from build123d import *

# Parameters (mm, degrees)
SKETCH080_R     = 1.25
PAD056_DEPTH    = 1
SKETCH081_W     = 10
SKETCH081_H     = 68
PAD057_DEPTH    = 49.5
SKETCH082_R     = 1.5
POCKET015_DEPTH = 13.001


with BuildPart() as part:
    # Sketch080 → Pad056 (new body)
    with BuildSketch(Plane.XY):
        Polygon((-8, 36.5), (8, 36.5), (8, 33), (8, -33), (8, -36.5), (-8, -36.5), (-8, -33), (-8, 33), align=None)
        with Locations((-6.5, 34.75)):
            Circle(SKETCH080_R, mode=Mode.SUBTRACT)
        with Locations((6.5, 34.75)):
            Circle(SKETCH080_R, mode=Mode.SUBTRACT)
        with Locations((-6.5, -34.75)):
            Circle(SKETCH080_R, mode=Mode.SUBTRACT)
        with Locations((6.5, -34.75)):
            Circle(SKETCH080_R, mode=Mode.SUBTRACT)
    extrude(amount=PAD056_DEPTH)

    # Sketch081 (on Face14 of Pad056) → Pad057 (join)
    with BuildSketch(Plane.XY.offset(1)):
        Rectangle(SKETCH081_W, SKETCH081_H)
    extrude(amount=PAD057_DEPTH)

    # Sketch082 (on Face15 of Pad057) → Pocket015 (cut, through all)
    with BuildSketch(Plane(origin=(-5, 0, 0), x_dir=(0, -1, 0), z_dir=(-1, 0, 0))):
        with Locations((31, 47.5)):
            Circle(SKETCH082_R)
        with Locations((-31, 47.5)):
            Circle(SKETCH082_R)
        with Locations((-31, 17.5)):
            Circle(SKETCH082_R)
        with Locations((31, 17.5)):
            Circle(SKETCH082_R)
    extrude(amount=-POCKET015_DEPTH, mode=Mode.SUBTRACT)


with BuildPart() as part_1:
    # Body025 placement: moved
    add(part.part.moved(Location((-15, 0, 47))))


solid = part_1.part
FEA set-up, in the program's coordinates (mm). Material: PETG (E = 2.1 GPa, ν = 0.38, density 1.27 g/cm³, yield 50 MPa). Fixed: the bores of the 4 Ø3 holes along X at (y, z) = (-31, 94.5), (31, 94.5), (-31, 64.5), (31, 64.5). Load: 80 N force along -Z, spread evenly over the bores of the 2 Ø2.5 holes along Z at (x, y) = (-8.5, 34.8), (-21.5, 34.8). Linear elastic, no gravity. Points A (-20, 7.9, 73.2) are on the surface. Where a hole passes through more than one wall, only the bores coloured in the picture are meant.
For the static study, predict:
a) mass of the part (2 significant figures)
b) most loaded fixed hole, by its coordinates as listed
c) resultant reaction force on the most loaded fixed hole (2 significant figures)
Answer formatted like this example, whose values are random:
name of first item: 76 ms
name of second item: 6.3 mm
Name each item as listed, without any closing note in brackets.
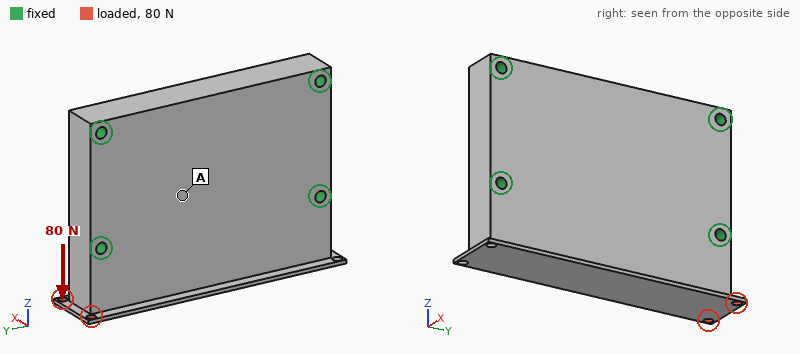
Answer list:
mass of the part: 44 g
most loaded fixed hole, by its coordinates as listed: (31, 64.5)
resultant reaction force on the most loaded fixed hole: 82 N
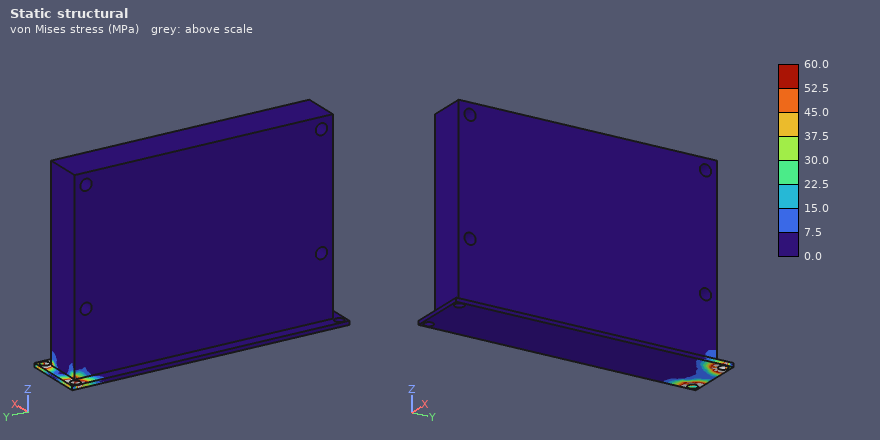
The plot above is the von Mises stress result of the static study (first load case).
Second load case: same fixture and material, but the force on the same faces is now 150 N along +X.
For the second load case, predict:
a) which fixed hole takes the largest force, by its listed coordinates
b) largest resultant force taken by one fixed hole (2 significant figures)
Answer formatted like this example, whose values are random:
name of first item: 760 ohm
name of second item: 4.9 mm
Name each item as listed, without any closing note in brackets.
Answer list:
which fixed hole takes the largest force, by its listed coordinates: (31, 64.5)
largest resultant force taken by one fixed hole: 190 N
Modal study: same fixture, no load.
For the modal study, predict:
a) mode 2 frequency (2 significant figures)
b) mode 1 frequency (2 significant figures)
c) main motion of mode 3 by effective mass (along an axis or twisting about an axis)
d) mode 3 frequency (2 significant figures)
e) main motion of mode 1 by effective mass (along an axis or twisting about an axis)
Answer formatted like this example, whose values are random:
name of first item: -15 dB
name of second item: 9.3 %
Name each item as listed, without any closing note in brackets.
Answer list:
mode 2 frequency: 2900 Hz
mode 1 frequency: 2200 Hz
main motion of mode 3 by effective mass: twisting about Z
mode 3 frequency: 4600 Hz
main motion of mode 1 by effective mass: along X
